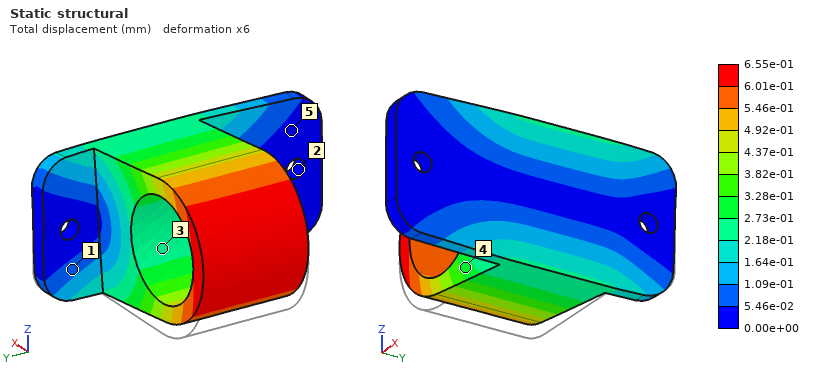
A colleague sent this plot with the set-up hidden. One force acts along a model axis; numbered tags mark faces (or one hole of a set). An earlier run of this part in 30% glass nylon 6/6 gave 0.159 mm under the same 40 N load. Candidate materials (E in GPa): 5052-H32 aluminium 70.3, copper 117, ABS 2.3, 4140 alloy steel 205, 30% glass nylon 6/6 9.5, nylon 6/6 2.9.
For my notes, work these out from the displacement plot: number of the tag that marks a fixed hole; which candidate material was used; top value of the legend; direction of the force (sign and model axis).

2
ABS
6.55e-01 mm
+Z
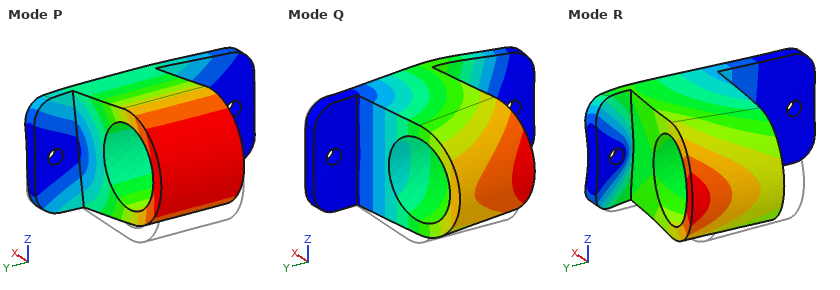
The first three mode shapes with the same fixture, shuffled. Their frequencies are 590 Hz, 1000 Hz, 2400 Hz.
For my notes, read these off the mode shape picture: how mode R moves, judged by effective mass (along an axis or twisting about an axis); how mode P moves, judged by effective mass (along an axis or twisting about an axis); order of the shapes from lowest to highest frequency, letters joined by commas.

along X
along Z
P, Q, R
